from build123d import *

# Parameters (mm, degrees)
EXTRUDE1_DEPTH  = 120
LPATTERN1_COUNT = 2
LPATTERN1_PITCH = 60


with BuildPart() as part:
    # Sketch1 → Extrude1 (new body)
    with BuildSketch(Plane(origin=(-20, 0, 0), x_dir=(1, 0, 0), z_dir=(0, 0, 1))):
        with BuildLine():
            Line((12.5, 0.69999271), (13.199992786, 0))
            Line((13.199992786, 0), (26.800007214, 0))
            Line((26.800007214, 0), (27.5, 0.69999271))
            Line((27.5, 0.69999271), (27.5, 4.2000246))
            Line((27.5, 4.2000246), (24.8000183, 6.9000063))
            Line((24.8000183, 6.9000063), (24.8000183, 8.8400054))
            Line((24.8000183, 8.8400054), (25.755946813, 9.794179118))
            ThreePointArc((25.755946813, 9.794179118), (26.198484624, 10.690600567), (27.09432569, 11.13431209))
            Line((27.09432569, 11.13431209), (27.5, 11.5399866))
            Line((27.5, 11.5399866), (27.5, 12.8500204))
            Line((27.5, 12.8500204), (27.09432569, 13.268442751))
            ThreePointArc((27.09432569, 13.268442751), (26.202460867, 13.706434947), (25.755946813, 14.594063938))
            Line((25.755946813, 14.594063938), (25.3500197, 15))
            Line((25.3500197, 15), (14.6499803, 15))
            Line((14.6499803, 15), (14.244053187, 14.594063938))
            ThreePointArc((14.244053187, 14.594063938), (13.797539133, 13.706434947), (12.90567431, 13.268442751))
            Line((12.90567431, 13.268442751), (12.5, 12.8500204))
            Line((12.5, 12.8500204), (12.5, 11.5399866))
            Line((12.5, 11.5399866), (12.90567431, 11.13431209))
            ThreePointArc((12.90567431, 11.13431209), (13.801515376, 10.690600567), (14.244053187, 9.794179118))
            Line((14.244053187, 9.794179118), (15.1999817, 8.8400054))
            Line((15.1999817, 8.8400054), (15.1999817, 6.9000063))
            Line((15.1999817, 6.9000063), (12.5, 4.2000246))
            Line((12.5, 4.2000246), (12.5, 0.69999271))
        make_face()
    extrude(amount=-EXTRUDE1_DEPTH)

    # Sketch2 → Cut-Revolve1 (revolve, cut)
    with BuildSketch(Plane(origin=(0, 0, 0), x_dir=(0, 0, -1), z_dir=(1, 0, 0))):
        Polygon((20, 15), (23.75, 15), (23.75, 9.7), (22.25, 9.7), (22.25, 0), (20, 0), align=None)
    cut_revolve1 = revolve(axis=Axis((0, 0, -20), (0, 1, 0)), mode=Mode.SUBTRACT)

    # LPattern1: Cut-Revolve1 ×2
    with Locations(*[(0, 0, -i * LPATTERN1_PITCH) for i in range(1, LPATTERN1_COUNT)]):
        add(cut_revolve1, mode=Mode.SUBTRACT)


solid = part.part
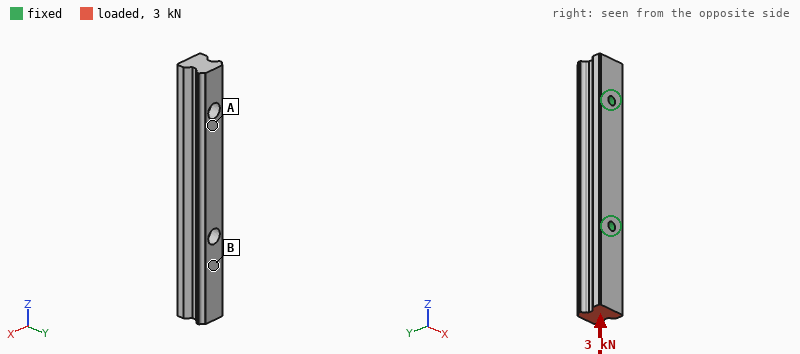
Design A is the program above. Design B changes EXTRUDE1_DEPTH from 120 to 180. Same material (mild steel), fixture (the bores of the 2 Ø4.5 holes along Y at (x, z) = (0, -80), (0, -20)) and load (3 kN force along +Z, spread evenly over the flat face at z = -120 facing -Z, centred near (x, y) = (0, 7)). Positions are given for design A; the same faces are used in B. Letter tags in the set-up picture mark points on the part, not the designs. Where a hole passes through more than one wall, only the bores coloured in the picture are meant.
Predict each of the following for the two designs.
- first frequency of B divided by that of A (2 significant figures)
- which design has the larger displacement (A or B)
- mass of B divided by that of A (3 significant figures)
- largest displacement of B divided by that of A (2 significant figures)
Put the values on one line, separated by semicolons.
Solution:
0.19; B; 1.52; 2.3
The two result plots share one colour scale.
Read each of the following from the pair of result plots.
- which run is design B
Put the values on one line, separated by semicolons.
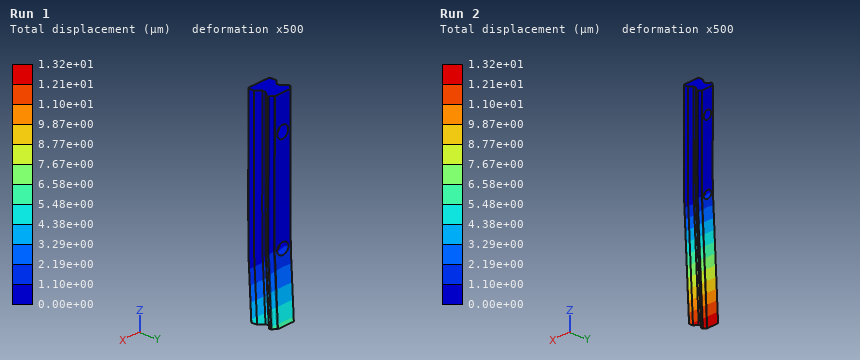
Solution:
Run 2
